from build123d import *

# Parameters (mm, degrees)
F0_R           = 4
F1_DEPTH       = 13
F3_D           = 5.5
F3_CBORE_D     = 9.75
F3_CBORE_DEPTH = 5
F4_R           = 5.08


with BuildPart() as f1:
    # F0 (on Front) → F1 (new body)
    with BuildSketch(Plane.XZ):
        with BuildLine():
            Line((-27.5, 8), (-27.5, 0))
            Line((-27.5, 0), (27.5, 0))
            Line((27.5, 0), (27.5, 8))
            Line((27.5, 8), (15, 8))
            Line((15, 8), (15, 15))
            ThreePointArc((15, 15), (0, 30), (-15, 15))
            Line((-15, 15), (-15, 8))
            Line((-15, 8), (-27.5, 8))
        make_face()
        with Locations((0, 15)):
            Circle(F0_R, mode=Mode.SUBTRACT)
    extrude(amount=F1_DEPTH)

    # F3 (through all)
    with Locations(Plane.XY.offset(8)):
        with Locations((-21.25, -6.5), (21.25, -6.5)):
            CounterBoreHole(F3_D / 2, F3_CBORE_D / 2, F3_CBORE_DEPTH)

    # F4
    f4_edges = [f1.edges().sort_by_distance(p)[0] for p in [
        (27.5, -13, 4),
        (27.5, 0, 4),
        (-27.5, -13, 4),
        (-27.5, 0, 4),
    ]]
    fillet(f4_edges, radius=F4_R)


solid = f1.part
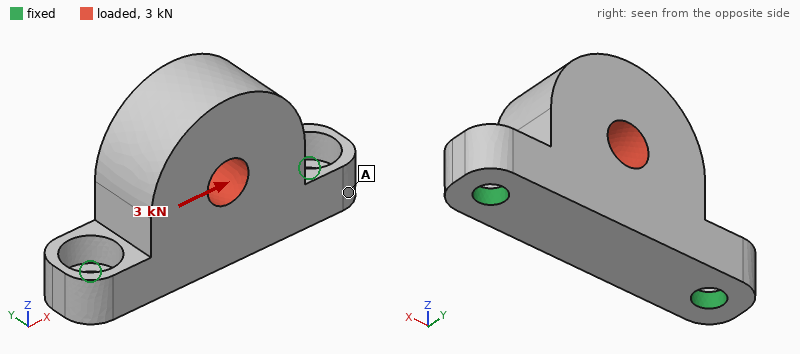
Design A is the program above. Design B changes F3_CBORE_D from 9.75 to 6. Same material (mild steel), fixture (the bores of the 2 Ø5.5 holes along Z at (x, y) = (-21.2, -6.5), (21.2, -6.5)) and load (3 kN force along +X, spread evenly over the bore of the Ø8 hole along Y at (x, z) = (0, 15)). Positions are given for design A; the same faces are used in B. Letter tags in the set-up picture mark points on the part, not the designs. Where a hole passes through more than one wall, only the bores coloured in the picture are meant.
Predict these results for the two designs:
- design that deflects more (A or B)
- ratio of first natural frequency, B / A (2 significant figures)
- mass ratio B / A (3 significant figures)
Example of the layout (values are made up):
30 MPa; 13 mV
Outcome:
A; 1.2; 1.04
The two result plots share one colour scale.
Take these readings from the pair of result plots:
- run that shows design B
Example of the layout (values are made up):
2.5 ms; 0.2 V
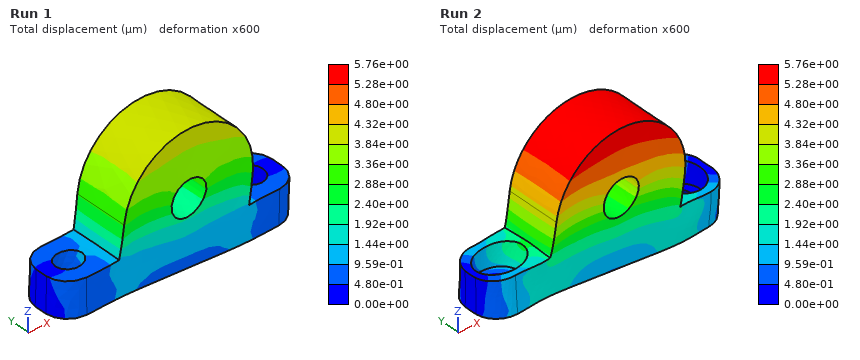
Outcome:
Run 1
